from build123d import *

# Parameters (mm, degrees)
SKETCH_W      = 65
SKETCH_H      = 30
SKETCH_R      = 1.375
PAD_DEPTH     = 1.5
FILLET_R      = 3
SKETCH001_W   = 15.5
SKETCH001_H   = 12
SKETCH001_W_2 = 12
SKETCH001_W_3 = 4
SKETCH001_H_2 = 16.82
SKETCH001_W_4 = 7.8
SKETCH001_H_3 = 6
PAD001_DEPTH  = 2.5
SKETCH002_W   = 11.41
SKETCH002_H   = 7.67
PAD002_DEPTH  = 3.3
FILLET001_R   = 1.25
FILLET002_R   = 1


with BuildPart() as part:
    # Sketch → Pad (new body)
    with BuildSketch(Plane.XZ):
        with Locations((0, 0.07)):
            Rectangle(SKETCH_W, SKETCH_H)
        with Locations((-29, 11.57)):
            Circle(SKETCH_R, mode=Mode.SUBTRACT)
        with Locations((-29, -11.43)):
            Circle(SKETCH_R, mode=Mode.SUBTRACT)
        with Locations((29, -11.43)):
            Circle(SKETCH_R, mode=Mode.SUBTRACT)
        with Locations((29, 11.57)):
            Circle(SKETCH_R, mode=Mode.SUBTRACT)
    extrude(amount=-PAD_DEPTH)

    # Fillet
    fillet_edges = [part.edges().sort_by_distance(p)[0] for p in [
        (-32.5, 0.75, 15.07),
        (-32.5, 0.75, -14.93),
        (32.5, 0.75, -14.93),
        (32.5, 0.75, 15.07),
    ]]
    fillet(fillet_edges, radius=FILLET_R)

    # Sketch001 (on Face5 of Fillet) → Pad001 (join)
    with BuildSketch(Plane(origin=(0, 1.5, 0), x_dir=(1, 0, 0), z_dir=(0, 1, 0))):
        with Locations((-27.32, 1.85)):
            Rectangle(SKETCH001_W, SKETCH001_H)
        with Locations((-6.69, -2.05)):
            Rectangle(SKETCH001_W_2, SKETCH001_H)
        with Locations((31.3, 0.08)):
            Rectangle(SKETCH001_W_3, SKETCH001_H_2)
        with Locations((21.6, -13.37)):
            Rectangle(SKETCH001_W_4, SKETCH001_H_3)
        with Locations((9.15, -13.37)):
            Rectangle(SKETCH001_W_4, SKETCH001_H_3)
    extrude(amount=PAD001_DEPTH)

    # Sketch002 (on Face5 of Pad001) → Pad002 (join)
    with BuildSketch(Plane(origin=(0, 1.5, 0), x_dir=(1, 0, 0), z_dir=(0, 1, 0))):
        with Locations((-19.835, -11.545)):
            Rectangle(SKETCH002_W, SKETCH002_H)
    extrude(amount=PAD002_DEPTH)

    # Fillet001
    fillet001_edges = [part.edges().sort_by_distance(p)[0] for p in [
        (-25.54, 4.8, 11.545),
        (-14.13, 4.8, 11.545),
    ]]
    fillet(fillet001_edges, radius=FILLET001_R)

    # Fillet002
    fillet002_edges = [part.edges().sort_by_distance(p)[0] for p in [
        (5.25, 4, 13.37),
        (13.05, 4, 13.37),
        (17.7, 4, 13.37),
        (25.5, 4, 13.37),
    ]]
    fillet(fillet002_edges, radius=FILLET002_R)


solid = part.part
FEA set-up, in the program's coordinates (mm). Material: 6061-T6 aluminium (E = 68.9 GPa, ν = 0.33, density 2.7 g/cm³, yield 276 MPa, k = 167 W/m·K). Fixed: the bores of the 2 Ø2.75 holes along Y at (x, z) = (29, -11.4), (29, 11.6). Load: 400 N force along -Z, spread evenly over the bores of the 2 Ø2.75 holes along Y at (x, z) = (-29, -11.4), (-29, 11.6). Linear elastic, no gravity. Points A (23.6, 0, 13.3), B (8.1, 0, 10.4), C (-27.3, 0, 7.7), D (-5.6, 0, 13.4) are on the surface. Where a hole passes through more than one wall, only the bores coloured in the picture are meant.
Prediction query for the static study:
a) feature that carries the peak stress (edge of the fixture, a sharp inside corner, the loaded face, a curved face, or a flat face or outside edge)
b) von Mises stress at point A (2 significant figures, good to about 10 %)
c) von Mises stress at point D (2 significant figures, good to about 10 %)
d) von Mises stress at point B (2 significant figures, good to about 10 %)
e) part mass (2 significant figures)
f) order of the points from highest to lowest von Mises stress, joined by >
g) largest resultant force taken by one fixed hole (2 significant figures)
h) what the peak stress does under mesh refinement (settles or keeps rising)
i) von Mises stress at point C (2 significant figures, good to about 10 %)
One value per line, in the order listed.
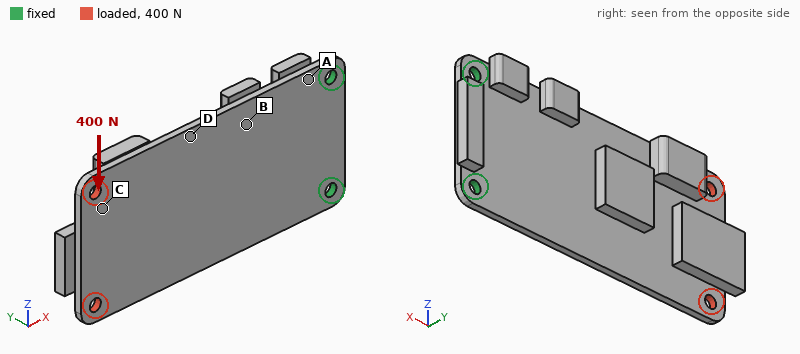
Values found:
edge of the fixture
91 MPa
37 MPa
53 MPa
12 g
A > B > D > C
1000 N
keeps rising
18 MPa
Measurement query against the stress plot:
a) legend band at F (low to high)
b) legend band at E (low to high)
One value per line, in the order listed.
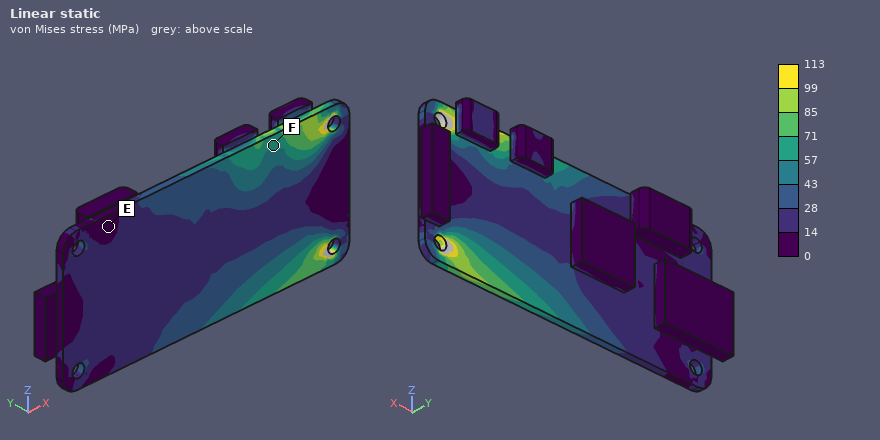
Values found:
57 to 71 MPa
0 to 14 MPa
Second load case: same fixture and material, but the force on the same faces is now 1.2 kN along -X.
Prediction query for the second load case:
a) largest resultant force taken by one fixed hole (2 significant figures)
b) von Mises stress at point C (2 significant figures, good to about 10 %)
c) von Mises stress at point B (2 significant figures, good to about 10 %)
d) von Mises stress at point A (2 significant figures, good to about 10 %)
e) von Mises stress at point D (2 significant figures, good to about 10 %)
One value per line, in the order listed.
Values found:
610 N
39 MPa
29 MPa
43 MPa
32 MPa
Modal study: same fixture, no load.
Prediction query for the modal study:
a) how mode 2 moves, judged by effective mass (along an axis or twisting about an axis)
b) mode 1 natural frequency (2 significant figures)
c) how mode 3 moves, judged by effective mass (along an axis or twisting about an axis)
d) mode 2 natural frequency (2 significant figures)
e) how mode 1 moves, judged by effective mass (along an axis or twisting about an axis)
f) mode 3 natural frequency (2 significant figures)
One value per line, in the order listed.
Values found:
twisting about X
270 Hz
along Y
1500 Hz
along Y
2100 Hz
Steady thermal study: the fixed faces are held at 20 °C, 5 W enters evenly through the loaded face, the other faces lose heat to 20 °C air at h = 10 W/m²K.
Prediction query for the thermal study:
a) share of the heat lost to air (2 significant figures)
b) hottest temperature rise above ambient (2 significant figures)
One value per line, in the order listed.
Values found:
16 %
34 K
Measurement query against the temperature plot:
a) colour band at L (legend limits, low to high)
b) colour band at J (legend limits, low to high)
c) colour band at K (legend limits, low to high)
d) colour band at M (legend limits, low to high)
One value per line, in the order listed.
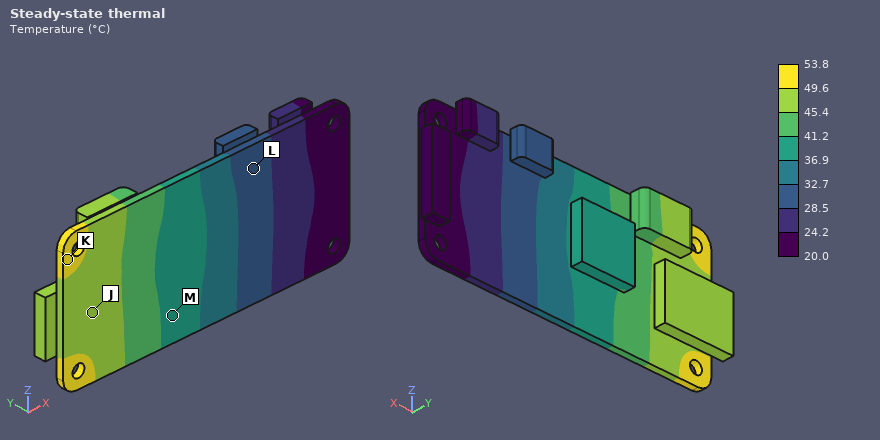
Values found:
28.5 to 32.7 °C
45.4 to 49.6 °C
49.6 to 53.8 °C
36.9 to 41.2 °C
